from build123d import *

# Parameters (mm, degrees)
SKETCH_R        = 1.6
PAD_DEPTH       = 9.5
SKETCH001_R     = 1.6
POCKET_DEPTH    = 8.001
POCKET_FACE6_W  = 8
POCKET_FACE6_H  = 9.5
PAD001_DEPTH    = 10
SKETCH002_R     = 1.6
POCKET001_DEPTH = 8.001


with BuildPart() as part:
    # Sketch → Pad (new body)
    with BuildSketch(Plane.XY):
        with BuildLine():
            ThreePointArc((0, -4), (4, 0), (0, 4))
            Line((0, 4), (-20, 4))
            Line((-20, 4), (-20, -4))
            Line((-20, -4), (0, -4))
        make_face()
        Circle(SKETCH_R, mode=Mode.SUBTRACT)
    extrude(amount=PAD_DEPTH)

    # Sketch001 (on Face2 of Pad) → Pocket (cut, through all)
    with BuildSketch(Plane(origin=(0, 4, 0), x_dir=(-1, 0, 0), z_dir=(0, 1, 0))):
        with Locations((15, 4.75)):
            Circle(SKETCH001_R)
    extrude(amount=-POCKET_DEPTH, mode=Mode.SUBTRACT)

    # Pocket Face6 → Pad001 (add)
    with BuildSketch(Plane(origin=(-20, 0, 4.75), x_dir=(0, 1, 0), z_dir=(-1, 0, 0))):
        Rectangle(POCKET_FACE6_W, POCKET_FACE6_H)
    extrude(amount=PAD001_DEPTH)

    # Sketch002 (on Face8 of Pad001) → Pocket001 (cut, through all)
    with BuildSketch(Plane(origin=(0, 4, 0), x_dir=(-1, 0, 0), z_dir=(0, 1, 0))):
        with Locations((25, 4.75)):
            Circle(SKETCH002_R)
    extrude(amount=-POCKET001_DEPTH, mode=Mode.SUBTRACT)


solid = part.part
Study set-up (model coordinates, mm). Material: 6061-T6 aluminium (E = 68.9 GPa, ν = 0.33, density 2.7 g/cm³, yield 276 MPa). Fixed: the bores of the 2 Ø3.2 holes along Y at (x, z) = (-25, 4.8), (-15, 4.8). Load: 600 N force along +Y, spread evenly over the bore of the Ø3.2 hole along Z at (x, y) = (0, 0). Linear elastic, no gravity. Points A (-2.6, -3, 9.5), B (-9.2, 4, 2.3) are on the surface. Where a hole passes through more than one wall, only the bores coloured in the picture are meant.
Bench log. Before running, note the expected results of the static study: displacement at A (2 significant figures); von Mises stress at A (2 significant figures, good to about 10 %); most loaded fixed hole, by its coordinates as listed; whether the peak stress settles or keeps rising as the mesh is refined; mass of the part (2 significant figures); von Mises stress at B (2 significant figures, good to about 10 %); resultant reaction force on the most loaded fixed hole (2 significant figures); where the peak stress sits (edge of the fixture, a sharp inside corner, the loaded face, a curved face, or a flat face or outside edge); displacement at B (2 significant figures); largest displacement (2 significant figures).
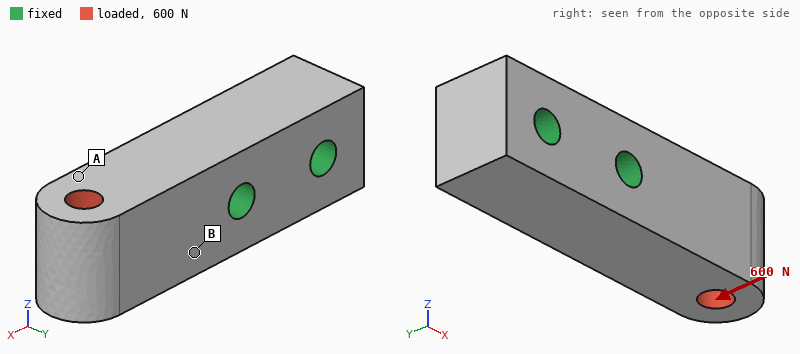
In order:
22 µm
15 MPa
(-15, 4.8)
keeps rising
6.2 g
54 MPa
710 N
edge of the fixture
8.8 µm
39 µm
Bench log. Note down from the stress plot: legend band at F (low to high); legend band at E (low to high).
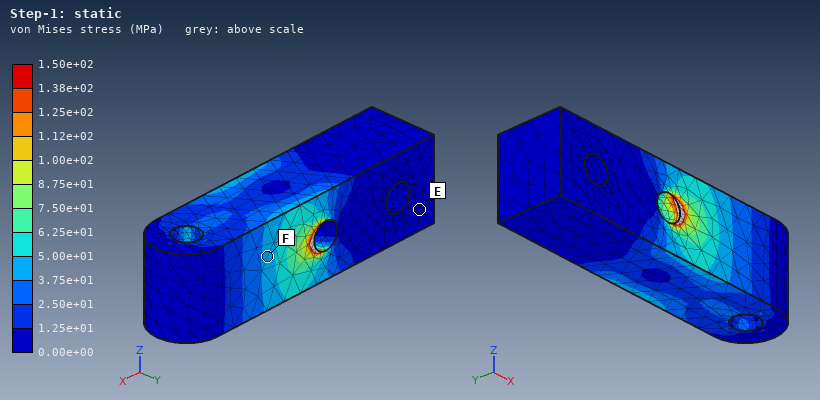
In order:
3.75e+01 to 5.00e+01 MPa
0.00e+00 to 1.25e+01 MPa
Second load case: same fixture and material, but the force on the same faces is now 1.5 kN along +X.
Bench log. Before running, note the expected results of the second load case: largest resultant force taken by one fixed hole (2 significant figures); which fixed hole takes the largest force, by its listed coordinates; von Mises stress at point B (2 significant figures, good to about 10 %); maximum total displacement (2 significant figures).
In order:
1.4 kN
(-15, 4.8)
20 MPa
6.1 µm
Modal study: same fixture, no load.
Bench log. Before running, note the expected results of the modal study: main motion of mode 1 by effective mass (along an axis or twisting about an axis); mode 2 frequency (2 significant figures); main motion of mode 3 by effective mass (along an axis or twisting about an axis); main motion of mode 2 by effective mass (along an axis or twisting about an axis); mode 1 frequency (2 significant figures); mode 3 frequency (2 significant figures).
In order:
along Z
19 kHz
twisting about X
along Y
18 kHz
41 kHz
